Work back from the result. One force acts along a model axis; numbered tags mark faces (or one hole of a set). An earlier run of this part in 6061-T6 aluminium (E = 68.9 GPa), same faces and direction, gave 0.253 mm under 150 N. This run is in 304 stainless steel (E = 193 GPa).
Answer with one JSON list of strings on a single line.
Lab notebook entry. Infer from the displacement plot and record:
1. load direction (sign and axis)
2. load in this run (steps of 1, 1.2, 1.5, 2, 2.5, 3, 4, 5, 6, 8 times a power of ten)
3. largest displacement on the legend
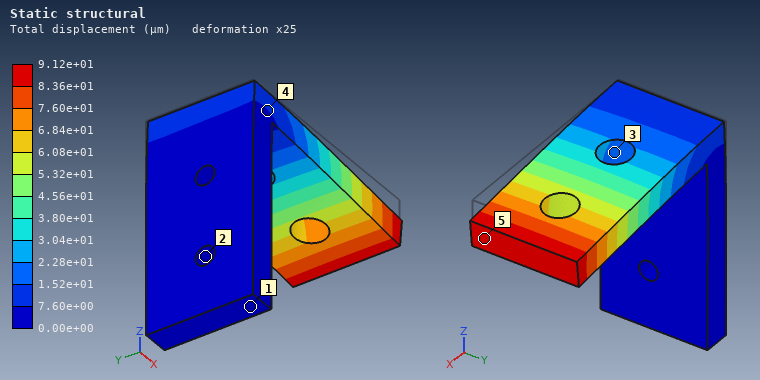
["-Z", "150 N", "9.12e+01 µm"]
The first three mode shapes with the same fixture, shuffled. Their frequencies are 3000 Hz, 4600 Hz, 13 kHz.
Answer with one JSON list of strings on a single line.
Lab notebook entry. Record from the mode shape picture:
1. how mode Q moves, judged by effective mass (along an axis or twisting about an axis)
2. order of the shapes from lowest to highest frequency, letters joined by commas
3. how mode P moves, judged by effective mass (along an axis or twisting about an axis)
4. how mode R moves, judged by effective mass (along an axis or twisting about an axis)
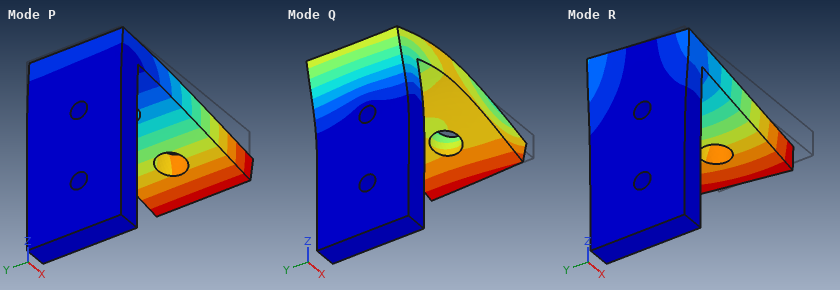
["along X", "P, R, Q", "along Z", "along Y"]
